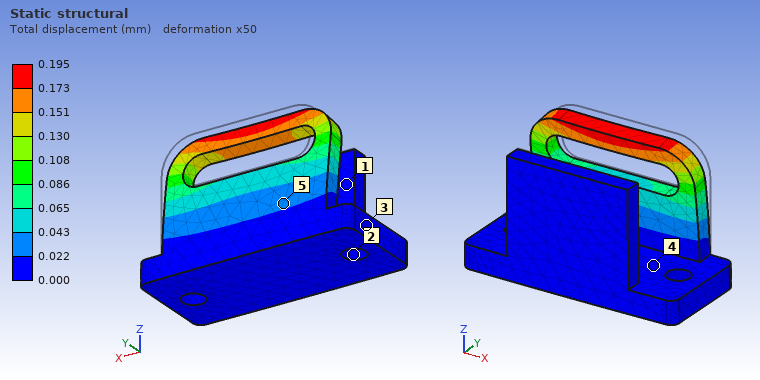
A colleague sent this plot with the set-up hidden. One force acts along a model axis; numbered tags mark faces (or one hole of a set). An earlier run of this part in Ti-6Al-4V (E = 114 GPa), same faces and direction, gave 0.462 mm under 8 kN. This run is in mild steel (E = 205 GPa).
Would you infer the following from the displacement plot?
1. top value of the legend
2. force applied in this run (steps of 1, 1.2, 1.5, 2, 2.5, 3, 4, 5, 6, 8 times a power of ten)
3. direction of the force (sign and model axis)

0.195 mm
6 kN
-Y
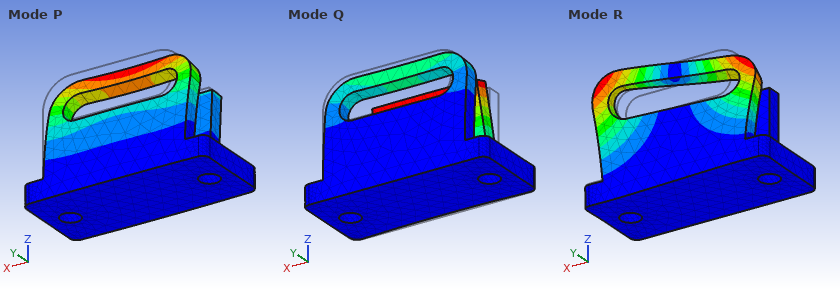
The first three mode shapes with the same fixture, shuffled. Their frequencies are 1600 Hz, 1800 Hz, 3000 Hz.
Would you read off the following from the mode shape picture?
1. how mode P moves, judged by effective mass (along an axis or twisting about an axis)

along Y
